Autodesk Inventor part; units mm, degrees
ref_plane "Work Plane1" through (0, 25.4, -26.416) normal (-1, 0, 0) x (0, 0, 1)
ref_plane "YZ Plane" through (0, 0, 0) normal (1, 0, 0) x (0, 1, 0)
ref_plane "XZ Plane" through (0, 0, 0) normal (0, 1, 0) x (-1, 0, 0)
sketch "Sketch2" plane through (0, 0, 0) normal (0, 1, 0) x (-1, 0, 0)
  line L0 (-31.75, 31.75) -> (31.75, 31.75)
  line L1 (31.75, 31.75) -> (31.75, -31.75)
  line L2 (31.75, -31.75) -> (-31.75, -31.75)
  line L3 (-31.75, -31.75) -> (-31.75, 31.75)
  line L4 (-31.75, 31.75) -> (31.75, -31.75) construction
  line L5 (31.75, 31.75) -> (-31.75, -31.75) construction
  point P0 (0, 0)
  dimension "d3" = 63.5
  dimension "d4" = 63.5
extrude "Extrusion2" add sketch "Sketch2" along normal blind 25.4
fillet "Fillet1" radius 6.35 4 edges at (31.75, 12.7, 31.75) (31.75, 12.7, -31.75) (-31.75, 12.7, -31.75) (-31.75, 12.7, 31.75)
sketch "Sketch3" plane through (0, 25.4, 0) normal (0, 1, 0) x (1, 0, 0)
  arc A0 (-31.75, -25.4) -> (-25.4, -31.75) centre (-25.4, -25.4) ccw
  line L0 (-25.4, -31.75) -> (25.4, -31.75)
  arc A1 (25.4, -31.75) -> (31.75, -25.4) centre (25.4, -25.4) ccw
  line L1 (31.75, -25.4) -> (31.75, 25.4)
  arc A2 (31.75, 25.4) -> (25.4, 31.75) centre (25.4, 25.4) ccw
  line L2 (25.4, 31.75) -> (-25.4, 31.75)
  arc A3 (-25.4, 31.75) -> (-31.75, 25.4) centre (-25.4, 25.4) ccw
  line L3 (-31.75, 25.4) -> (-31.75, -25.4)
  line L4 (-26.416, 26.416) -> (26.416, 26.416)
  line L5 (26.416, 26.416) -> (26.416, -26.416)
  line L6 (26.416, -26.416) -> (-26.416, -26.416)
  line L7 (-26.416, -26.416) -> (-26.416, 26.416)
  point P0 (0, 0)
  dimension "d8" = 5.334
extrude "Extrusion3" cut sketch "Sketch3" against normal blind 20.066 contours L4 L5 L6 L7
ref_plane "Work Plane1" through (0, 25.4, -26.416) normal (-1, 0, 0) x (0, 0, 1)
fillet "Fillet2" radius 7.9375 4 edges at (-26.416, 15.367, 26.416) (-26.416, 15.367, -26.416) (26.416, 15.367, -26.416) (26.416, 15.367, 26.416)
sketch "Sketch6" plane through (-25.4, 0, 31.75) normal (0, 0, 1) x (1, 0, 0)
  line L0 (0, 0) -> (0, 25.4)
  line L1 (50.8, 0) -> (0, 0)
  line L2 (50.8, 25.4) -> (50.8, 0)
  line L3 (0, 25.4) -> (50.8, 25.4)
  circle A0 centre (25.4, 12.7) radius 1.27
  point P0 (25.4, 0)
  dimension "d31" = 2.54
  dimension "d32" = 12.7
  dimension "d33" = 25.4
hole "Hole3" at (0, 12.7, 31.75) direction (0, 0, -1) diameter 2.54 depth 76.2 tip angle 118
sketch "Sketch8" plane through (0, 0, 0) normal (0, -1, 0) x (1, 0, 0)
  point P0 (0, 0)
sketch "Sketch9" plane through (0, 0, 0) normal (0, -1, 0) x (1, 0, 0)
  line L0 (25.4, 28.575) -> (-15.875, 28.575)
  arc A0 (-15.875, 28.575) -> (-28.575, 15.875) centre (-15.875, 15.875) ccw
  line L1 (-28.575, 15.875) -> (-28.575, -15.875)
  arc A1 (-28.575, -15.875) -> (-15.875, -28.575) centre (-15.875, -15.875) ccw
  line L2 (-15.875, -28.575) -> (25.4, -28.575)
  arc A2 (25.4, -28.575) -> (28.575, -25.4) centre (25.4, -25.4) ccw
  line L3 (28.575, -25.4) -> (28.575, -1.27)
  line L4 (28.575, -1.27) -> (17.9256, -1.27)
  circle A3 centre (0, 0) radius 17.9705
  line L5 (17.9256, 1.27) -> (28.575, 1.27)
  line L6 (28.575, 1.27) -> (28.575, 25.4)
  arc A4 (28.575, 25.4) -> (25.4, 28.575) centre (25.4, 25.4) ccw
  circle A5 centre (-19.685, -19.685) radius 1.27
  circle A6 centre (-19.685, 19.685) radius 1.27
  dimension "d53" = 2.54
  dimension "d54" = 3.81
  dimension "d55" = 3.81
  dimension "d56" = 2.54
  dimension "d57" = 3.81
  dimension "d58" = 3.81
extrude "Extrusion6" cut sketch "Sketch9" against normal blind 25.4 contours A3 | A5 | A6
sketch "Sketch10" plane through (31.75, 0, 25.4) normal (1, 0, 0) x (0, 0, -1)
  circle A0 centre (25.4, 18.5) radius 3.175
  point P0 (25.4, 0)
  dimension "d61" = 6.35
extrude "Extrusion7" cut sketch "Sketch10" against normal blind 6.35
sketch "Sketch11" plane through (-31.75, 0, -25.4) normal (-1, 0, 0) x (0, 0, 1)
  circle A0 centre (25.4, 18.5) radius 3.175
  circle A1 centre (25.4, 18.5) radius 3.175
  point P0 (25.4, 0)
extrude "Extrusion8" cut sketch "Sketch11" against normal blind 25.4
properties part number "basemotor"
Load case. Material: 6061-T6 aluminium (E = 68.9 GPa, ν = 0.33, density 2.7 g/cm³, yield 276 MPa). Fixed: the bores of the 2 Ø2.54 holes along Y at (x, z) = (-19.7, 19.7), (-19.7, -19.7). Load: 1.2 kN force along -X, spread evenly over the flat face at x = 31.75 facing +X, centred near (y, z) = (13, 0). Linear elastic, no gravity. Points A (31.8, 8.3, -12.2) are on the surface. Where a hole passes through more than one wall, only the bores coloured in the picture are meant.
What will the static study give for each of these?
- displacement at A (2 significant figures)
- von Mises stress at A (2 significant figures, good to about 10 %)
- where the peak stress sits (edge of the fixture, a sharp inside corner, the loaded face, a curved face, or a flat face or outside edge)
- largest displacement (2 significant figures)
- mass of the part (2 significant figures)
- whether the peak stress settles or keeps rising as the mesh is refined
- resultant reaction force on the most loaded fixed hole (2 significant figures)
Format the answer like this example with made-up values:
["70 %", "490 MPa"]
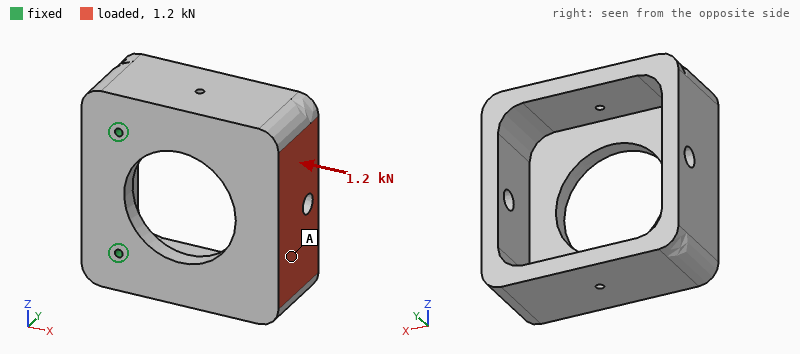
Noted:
["0.11 mm", "11 MPa", "edge of the fixture", "0.13 mm", "110 g", "keeps rising", "680 N"]
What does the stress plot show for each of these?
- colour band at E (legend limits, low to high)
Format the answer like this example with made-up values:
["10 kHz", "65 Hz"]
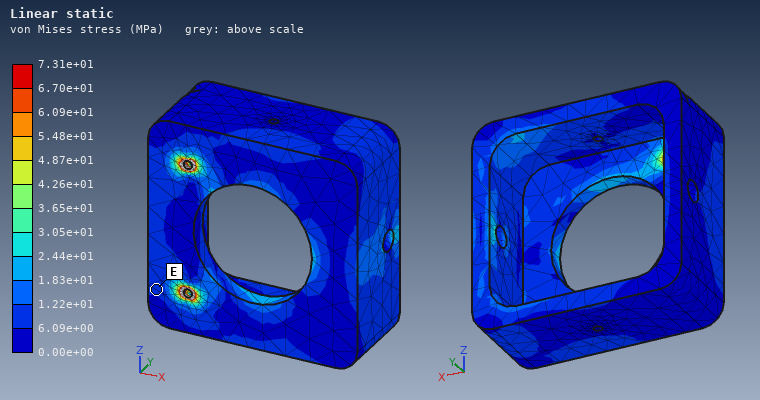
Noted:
["6.09e+00 to 1.22e+01 MPa"]
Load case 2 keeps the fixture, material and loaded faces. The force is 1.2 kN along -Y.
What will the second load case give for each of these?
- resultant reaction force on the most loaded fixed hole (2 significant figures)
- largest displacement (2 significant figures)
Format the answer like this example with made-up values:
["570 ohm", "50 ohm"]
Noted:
["740 N", "0.59 mm"]
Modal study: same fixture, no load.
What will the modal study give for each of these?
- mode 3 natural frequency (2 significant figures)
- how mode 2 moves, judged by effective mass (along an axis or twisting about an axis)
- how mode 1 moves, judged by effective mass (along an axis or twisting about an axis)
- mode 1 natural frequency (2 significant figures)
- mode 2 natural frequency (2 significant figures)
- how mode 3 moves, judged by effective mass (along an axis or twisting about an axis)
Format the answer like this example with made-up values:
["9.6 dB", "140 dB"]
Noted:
["3600 Hz", "along Z", "along Y", "1200 Hz", "2500 Hz", "along Z"]
